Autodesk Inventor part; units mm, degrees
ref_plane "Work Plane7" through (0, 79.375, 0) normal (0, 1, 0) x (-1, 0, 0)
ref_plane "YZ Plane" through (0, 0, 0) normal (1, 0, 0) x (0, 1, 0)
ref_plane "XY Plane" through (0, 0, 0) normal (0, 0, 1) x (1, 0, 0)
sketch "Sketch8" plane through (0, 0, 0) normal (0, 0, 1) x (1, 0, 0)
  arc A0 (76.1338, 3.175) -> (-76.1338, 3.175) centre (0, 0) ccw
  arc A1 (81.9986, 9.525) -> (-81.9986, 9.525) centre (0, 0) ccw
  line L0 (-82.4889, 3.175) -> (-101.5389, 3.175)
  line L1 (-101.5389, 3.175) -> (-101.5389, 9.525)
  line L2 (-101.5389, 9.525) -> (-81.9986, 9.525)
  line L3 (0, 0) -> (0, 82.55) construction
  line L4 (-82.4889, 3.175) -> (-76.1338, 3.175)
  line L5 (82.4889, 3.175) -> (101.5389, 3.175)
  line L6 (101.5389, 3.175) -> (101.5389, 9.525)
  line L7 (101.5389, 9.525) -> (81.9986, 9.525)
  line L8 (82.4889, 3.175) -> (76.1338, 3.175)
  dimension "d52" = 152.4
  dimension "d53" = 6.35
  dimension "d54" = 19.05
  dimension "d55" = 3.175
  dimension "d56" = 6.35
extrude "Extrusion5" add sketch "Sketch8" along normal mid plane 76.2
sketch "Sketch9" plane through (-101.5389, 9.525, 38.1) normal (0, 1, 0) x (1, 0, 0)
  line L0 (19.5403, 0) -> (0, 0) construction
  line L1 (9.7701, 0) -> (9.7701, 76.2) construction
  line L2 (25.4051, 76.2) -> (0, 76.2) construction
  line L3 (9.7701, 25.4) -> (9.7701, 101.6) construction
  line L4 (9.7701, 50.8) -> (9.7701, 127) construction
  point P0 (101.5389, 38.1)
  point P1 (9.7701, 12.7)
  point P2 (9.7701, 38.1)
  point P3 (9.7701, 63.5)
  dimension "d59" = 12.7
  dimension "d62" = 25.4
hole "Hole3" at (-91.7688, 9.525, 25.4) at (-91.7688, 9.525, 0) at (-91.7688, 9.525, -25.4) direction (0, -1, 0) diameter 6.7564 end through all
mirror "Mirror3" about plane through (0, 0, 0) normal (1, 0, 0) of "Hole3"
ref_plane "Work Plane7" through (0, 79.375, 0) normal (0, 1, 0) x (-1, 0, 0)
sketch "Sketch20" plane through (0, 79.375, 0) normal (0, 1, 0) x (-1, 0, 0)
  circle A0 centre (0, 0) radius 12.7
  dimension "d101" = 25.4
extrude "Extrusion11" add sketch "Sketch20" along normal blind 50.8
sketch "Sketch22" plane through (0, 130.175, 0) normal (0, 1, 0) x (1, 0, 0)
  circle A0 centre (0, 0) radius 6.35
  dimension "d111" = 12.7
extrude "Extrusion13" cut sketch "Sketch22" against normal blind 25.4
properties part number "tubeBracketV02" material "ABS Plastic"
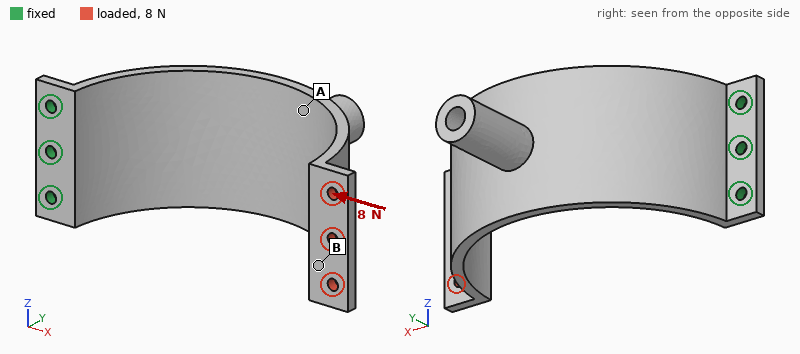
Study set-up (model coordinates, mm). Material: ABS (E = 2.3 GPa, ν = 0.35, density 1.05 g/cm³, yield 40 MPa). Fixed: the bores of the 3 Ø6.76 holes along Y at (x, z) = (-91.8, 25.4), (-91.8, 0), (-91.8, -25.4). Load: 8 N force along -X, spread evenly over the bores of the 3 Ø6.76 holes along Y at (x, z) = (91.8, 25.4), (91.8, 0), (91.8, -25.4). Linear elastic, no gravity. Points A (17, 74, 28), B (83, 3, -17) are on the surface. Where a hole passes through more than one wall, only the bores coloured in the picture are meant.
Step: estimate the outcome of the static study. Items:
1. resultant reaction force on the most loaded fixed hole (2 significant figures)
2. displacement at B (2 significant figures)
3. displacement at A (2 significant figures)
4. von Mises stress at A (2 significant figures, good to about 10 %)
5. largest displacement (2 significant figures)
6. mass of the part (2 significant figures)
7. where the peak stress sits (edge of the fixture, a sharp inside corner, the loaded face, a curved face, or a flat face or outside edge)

3.6 N
2.1 mm
0.62 mm
0.96 MPa
2.5 mm
160 g
a curved face
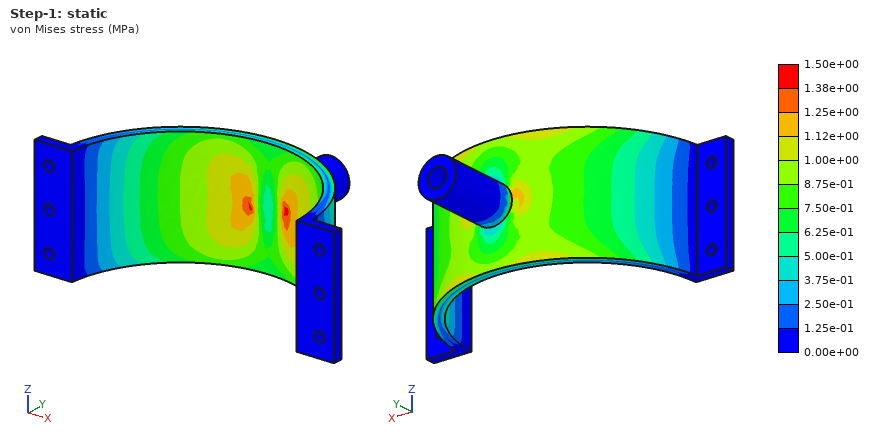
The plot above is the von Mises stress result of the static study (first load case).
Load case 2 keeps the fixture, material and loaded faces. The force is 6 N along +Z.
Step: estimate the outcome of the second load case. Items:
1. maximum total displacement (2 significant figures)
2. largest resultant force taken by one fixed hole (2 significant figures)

2.3 mm
20 N
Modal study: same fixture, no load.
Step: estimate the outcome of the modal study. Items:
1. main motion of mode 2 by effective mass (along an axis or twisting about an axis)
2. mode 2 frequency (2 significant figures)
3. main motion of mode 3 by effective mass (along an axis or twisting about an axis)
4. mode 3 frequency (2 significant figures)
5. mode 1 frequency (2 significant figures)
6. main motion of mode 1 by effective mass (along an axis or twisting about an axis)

along Z
46 Hz
along X
83 Hz
26 Hz
along Y
